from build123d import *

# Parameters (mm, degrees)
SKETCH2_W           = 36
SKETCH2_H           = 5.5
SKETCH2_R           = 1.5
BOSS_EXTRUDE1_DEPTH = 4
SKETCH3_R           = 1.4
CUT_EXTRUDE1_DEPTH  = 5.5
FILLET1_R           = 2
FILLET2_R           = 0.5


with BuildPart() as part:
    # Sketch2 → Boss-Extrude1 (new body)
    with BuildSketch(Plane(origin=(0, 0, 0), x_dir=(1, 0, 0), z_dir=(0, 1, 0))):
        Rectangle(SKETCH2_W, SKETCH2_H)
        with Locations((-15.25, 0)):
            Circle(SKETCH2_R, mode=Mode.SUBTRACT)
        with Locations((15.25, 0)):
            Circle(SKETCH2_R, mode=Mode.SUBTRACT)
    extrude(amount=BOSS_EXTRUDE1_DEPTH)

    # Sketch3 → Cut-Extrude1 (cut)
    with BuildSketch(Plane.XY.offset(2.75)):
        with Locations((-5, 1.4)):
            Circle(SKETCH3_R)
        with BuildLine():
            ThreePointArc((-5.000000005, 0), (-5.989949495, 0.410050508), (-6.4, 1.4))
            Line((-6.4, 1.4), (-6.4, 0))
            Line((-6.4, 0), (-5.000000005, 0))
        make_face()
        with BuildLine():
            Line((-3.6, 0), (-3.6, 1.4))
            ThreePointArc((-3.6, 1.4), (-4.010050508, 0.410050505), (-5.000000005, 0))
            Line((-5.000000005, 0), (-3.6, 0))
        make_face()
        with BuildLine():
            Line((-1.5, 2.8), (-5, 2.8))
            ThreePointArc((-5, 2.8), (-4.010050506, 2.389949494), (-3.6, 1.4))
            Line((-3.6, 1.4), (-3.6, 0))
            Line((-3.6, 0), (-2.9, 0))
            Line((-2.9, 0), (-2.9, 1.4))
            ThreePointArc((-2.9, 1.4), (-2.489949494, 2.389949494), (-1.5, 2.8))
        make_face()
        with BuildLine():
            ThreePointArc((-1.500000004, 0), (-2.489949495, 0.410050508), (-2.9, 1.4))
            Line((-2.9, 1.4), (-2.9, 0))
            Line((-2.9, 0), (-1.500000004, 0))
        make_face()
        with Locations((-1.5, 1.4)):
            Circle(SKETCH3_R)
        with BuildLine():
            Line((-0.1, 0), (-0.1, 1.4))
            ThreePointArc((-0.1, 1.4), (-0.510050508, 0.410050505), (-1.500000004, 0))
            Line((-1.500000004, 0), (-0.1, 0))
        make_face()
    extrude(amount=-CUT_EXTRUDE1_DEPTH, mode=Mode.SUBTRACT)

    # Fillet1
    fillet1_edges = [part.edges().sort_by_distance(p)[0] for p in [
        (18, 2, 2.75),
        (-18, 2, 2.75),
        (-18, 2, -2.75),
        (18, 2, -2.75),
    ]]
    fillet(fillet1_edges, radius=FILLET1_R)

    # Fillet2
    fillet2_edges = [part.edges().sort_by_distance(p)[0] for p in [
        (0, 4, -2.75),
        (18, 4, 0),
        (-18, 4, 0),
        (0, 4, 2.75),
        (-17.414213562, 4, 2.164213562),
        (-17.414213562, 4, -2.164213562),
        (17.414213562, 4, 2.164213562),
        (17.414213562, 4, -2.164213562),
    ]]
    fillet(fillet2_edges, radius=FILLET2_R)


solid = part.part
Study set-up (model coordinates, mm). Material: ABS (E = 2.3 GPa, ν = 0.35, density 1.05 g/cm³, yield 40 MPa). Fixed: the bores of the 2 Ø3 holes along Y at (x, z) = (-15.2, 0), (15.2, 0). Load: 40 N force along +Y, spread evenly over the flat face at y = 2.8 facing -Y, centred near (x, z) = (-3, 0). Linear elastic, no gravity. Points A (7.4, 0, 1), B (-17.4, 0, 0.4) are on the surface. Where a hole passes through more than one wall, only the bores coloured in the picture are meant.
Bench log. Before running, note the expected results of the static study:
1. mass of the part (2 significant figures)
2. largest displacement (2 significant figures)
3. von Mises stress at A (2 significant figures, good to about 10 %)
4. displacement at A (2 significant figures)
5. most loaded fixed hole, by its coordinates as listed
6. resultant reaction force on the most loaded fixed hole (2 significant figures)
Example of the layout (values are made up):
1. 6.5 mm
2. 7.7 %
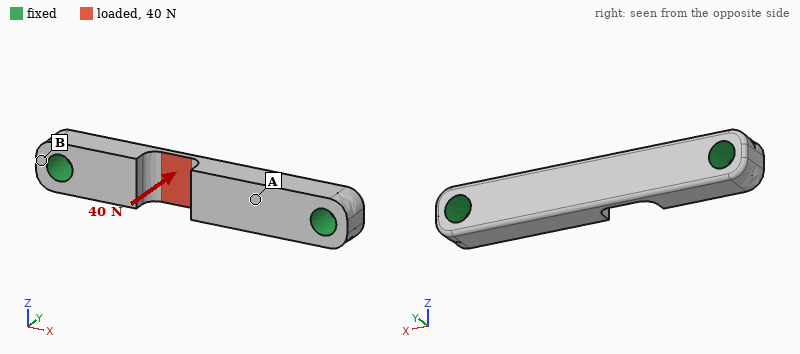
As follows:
1. 0.66 g
2. 0.17 mm
3. 5.5 MPa
4. 0.056 mm
5. (-15.2, 0)
6. 46 N
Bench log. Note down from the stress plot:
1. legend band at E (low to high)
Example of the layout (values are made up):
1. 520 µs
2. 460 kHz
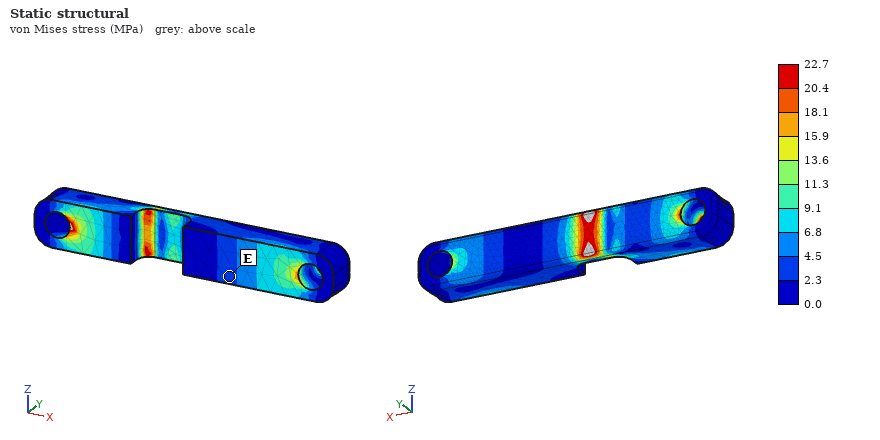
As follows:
1. 2.3 to 4.5 MPa
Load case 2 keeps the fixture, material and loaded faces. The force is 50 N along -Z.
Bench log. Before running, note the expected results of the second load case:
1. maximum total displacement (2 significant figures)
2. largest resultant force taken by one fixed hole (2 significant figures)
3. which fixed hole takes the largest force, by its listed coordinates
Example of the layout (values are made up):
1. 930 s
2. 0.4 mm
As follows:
1. 0.12 mm
2. 34 N
3. (-15.2, 0)
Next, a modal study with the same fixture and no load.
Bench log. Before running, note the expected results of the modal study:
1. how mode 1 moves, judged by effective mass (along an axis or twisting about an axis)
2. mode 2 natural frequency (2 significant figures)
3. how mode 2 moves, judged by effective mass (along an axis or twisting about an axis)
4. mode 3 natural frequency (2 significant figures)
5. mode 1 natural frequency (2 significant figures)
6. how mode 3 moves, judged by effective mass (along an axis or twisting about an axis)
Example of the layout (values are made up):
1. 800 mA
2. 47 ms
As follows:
1. along Y
2. 7700 Hz
3. along Z
4. 13 kHz
5. 6100 Hz
6. twisting about X
